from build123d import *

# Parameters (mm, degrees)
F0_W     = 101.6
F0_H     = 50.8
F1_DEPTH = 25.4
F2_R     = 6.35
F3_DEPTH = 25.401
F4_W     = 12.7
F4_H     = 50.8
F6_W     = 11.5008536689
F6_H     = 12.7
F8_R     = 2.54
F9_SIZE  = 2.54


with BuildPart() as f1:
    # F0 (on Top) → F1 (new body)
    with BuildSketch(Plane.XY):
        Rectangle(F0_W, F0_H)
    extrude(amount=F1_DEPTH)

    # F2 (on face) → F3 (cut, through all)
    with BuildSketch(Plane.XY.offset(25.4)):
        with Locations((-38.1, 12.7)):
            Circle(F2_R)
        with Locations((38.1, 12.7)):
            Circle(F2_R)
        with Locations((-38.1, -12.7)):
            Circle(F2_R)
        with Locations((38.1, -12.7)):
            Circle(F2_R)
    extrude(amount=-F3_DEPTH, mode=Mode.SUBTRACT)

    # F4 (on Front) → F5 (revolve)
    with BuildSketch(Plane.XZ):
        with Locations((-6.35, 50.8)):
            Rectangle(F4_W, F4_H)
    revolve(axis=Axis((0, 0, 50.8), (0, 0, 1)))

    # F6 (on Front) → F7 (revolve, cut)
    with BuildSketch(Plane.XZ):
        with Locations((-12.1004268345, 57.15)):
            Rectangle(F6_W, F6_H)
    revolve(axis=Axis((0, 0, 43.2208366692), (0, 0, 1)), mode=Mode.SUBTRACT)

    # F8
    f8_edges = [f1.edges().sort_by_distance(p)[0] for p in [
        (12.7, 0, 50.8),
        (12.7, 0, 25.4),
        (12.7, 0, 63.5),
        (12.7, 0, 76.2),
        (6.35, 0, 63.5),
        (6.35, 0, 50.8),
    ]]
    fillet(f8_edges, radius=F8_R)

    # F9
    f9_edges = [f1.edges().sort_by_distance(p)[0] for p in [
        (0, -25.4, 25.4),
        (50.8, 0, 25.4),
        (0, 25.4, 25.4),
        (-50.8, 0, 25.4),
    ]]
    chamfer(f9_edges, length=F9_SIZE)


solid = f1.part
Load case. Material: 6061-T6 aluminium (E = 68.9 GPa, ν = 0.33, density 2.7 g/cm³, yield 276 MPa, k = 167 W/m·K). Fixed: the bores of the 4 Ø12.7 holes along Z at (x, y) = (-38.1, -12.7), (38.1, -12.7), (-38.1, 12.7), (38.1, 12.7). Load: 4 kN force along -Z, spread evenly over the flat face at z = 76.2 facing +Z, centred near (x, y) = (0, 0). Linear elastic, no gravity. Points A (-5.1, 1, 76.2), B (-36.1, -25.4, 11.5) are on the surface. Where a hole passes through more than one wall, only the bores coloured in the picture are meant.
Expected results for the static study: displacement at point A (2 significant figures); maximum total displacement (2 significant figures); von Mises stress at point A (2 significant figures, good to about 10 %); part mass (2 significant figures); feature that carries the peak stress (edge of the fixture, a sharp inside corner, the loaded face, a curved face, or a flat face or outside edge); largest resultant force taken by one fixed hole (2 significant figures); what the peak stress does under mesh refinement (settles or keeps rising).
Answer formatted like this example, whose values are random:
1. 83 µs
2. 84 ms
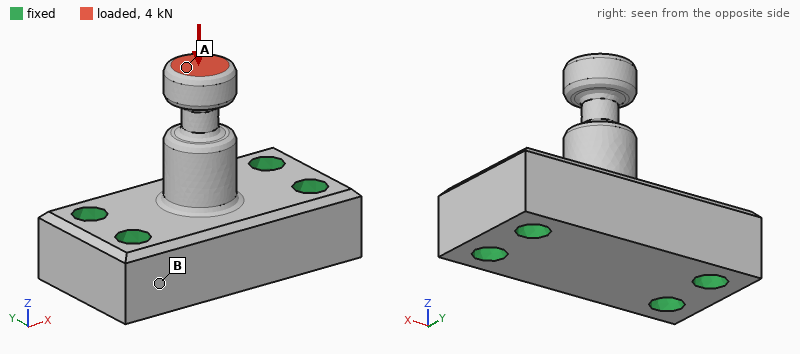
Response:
1. 15 µm
2. 15 µm
3. 11 MPa
4. 370 g
5. a sharp inside corner
6. 1.0 kN
7. keeps rising
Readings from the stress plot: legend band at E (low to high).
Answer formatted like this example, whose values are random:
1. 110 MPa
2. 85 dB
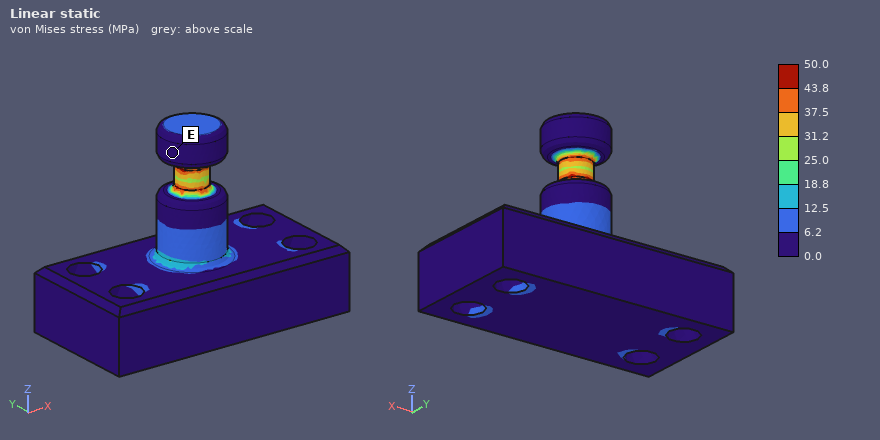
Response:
1. 0.0 to 6.2 MPa
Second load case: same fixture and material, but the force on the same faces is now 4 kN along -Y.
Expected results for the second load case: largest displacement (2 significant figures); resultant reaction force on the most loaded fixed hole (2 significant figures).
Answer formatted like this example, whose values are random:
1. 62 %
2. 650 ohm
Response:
1. 0.48 mm
2. 3.3 kN
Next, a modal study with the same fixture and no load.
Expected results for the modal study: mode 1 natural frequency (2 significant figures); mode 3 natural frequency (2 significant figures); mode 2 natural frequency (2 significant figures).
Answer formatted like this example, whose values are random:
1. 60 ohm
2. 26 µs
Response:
1. 4300 Hz
2. 8800 Hz
3. 4400 Hz
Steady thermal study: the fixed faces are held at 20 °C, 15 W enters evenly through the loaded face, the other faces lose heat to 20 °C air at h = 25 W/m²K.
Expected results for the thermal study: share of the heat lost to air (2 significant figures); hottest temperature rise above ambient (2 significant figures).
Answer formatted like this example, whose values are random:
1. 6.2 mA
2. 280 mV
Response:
1. 7.0 %
2. 19 K
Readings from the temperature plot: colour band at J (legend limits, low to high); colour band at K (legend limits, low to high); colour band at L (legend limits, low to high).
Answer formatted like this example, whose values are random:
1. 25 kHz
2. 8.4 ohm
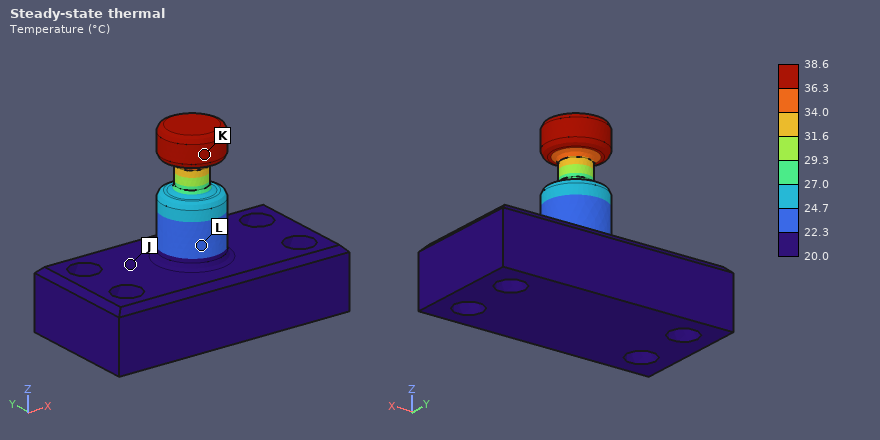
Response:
1. 20.0 to 22.3 °C
2. 36.3 to 38.6 °C
3. 22.3 to 24.7 °C
